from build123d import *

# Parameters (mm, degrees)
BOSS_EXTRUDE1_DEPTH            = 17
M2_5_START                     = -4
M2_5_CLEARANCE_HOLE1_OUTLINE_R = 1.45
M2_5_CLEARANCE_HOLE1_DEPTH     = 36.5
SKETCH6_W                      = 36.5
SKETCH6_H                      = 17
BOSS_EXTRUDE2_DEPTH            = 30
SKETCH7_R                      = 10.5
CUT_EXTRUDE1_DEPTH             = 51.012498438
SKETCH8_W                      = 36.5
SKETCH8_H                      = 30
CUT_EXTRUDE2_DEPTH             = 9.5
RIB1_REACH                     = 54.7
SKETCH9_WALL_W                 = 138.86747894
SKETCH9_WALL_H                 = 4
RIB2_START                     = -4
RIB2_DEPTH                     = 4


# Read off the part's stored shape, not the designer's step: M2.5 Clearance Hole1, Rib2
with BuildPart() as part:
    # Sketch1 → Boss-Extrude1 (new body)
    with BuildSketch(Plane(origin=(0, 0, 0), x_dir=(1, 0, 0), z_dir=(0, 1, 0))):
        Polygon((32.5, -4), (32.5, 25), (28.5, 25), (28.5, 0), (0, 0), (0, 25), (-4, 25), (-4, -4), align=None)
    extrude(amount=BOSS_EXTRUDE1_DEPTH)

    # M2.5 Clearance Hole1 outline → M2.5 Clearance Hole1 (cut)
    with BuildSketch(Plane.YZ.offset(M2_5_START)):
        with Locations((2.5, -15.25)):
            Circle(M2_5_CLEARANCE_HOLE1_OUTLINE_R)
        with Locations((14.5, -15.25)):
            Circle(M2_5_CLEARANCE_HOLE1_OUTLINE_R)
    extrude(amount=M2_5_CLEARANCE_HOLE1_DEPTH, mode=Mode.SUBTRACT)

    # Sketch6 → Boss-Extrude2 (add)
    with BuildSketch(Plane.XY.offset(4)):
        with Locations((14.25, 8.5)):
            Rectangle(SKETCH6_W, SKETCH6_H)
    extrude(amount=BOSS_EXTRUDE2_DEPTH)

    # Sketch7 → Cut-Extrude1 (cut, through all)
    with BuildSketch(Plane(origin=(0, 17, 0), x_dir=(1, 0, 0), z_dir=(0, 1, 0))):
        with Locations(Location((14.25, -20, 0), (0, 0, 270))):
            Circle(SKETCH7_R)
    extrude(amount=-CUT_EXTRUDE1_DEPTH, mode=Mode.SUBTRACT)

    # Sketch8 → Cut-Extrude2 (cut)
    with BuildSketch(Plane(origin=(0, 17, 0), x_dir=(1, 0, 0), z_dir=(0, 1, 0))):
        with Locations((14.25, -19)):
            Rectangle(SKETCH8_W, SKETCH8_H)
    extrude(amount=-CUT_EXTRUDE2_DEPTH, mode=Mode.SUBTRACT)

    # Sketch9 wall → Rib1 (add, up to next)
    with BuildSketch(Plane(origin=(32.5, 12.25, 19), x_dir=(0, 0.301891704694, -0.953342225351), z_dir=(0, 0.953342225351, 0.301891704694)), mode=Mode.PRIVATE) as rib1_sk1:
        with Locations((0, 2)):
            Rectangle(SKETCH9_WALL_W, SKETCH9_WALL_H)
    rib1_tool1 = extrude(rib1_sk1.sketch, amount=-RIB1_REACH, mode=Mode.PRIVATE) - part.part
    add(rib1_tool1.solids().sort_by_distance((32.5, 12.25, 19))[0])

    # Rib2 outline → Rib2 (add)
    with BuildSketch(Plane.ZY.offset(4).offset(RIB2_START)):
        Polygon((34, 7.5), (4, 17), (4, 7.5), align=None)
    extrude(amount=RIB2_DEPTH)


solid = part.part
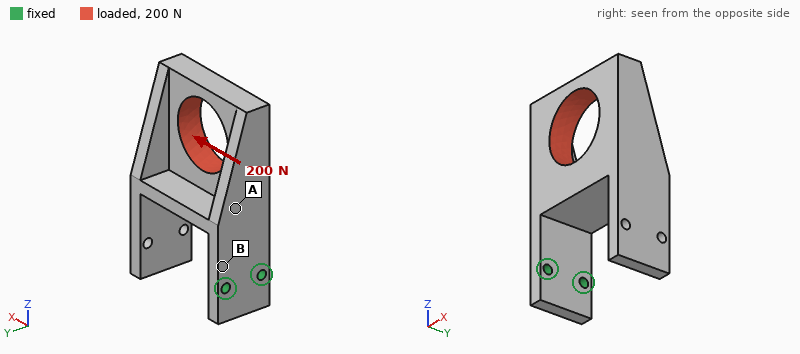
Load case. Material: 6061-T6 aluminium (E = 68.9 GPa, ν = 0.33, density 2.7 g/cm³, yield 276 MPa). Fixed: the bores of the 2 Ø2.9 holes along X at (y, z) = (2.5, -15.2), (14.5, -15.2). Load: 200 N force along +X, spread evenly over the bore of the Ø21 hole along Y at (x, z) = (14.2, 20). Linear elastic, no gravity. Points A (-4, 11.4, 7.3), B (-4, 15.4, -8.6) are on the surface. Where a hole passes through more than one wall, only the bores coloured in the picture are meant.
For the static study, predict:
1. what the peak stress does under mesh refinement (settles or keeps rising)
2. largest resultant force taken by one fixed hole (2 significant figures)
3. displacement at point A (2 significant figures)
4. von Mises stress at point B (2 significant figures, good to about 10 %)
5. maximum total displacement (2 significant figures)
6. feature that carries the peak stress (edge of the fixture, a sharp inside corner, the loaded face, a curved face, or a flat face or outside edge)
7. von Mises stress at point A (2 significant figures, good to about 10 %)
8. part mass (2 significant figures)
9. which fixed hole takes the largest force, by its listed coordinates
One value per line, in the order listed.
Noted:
keeps rising
170 N
0.21 mm
130 MPa
0.79 mm
edge of the fixture
19 MPa
34 g
(2.5, -15.2)
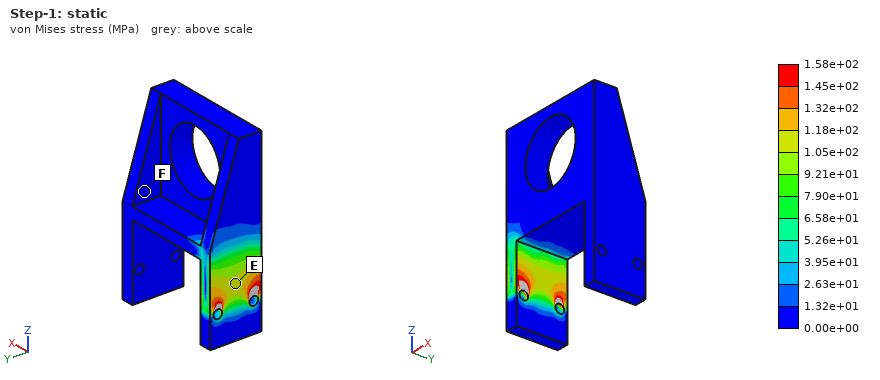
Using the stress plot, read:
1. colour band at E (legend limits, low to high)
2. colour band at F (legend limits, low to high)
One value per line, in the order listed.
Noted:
1.05e+02 to 1.18e+02 MPa
0.00e+00 to 1.32e+01 MPa
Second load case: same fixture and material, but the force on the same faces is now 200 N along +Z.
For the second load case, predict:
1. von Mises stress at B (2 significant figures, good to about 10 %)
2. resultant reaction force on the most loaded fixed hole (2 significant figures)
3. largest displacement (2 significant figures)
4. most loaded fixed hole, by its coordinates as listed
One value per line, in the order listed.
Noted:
74 MPa
180 N
0.48 mm
(2.5, -15.2)
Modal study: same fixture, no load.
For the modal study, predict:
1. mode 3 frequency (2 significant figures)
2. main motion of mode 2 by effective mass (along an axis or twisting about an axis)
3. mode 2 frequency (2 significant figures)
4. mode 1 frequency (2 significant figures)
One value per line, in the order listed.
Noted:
2800 Hz
along Y
1100 Hz
570 Hz
